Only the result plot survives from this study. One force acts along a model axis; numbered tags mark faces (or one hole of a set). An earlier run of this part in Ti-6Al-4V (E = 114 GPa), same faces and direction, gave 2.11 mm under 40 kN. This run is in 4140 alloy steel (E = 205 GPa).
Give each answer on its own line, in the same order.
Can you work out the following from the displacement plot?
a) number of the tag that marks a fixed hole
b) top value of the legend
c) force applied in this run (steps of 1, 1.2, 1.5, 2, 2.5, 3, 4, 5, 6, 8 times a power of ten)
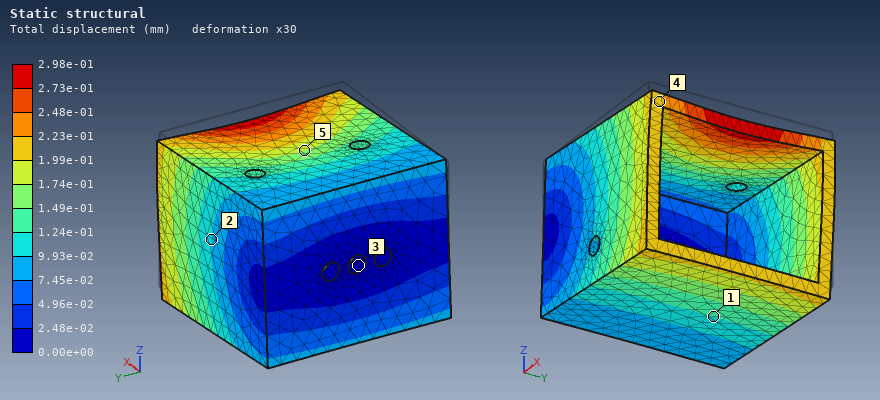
3
2.98e-01 mm
10 kN
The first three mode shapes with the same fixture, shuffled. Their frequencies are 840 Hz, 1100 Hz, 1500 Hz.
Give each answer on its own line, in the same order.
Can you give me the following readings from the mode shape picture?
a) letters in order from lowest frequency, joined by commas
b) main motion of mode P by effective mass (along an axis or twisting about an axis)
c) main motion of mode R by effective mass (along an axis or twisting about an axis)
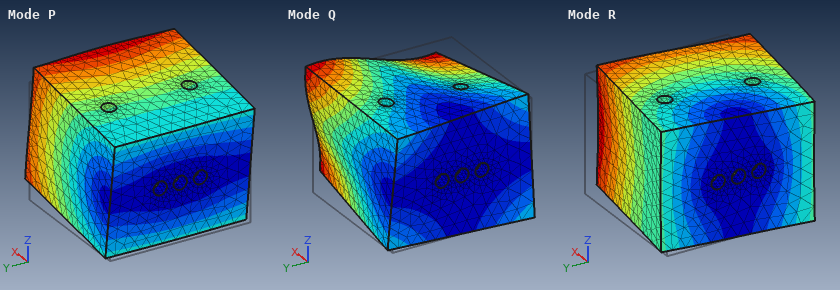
P, R, Q
along Z
along Y
